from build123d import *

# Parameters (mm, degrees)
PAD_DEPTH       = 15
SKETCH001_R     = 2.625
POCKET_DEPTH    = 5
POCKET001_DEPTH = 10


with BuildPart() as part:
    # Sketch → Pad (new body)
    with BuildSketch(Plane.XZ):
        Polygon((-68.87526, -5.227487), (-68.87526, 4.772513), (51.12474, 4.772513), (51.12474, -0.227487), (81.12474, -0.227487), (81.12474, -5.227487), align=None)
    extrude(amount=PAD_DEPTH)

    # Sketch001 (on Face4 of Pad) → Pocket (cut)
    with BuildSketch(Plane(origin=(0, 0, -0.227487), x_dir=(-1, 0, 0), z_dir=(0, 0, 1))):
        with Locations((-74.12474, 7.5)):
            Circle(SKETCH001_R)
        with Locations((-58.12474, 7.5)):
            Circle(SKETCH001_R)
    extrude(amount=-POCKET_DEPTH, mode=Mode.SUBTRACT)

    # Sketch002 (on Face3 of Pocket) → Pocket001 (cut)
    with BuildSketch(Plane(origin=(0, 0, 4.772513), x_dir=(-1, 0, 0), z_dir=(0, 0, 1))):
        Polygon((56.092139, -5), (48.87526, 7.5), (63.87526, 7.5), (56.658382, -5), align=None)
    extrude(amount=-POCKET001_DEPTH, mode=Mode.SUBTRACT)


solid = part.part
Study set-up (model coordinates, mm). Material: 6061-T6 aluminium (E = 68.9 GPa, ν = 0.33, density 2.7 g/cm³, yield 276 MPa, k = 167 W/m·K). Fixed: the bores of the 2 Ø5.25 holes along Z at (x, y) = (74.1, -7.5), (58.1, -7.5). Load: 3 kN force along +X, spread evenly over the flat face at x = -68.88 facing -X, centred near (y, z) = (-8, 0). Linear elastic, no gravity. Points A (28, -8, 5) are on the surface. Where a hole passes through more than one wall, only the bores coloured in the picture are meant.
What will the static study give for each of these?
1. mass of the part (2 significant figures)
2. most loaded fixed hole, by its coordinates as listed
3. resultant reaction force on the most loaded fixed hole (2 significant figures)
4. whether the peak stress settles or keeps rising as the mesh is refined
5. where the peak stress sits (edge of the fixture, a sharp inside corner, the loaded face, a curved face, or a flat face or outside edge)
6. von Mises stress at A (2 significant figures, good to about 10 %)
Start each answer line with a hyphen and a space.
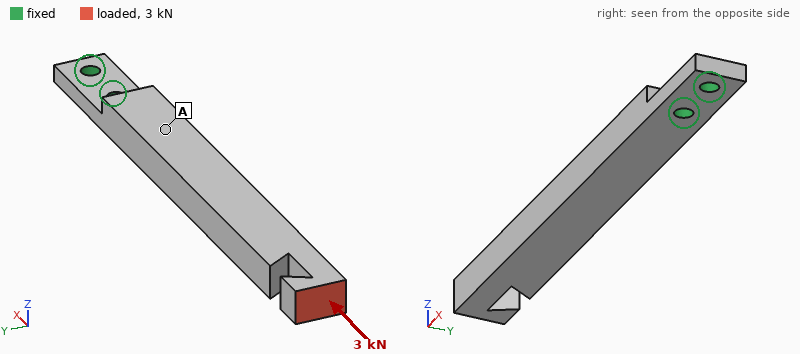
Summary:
- 52 g
- (58.1, -7.5)
- 2.7 kN
- keeps rising
- edge of the fixture
- 20 MPa
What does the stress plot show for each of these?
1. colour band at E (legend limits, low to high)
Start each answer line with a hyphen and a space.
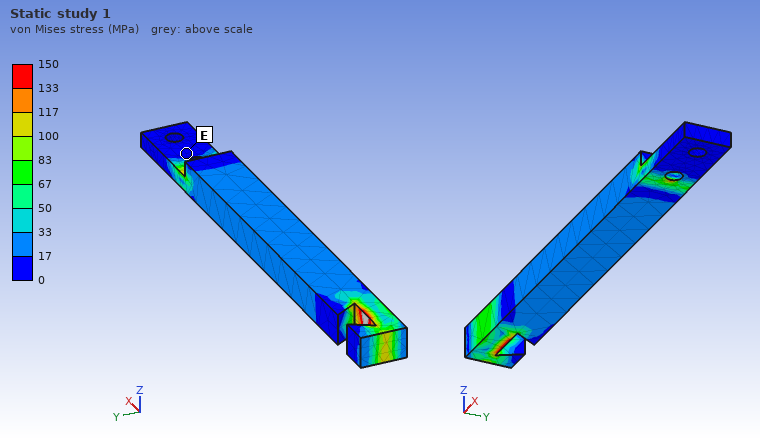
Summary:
- 0 to 17 MPa
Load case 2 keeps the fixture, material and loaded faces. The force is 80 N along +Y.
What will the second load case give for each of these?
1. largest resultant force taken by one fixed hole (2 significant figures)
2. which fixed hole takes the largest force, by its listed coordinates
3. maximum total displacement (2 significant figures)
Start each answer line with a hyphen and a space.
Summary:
- 350 N
- (58.1, -7.5)
- 0.42 mm
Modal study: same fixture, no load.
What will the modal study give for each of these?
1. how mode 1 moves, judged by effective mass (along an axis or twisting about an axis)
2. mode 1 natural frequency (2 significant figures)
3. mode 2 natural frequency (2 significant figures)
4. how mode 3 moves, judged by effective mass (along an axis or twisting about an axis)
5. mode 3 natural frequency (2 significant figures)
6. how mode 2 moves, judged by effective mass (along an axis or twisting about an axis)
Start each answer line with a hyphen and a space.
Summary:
- along Z
- 340 Hz
- 640 Hz
- along Z
- 2600 Hz
- along Y
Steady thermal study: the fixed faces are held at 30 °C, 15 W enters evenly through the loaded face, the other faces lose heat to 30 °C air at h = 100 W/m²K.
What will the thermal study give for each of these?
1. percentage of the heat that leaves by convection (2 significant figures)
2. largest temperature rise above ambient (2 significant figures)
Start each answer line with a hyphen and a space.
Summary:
- 73 %
- 50 K
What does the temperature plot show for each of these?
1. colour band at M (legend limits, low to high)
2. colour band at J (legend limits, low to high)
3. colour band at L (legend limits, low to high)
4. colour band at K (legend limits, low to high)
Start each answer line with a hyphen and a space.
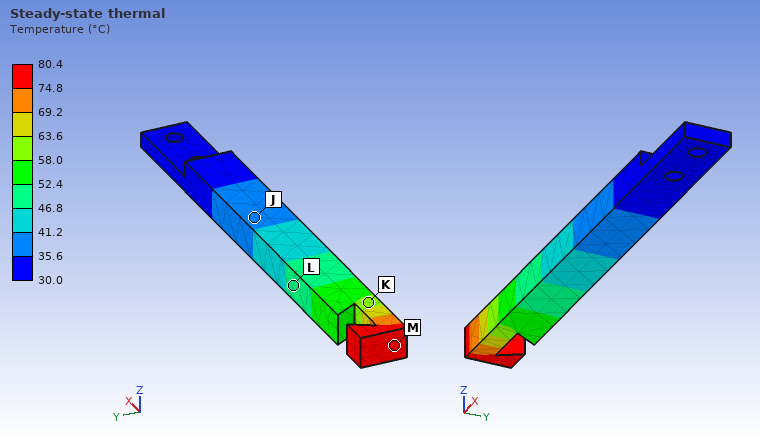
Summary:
- 74.8 to 80.4 °C
- 35.6 to 41.2 °C
- 46.8 to 52.4 °C
- 58.0 to 63.6 °C
